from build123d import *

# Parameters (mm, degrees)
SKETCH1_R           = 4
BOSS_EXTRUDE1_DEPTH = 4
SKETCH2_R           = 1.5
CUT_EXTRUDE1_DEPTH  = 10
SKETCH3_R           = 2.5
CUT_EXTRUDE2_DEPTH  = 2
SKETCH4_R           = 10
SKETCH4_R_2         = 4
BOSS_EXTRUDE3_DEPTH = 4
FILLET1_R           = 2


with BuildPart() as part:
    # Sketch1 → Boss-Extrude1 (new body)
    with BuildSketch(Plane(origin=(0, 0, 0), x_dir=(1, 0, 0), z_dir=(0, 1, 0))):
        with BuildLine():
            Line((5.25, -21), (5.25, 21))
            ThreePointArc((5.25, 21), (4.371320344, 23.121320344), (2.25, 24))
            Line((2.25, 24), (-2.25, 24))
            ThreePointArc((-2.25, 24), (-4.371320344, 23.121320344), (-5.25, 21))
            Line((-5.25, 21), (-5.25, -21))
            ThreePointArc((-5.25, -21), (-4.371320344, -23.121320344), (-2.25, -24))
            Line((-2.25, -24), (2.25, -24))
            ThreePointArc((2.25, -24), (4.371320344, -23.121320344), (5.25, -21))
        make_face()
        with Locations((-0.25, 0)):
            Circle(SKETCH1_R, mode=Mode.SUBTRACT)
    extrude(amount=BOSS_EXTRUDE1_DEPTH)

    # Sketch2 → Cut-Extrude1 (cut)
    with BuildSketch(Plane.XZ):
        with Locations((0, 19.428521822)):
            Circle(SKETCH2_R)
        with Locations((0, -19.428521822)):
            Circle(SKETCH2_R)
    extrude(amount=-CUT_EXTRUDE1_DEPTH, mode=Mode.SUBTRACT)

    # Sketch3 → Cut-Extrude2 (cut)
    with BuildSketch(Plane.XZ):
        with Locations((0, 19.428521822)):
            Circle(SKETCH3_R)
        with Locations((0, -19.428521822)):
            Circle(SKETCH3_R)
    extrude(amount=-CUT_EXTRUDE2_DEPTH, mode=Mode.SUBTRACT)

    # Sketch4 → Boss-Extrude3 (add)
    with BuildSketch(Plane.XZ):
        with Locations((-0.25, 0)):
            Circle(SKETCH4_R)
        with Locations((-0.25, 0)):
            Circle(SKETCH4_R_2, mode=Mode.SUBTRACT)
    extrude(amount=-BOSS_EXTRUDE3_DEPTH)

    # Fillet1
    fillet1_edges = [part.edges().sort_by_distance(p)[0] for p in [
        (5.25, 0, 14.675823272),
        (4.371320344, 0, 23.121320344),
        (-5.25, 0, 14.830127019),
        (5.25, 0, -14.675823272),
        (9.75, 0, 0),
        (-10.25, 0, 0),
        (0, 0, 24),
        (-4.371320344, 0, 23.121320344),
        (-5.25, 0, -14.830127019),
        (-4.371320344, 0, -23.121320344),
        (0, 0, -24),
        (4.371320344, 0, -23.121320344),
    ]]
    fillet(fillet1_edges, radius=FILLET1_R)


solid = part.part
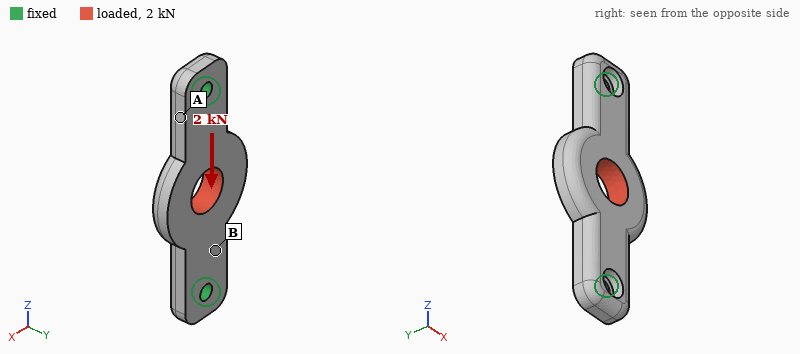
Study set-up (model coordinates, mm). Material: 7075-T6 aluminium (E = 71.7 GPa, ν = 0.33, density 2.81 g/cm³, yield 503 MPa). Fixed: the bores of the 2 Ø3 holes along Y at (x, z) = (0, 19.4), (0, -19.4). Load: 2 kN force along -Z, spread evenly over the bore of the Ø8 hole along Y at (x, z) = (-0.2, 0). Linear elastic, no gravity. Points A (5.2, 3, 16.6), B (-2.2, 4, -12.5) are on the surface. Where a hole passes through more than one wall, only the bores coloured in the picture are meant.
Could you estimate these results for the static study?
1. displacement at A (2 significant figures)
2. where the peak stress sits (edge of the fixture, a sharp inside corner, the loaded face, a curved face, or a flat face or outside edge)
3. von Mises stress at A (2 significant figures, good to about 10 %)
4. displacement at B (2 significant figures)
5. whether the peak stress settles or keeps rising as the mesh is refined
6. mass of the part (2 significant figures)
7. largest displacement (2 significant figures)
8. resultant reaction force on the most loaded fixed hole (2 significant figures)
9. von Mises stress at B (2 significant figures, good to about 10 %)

3.4 µm
edge of the fixture
16 MPa
4.6 µm
keeps rising
5.7 g
9.2 µm
1.0 kN
40 MPa
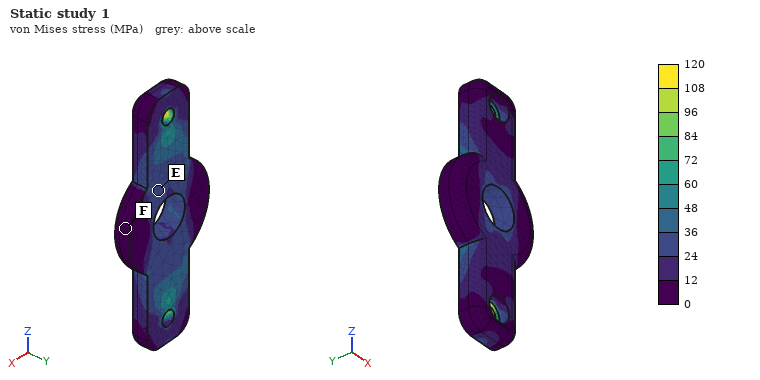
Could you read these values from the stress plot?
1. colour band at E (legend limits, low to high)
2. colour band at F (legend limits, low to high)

24 to 36 MPa
0 to 12 MPa
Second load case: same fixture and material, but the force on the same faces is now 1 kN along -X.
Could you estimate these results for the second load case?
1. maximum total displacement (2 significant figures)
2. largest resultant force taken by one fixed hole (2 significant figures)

23 µm
500 N
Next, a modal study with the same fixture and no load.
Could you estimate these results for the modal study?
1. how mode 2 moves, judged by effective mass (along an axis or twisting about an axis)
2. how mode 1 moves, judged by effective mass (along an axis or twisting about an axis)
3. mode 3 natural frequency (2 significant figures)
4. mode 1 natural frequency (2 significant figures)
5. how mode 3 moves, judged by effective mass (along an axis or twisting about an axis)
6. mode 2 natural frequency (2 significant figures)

twisting about Z
along Y
20 kHz
9000 Hz
along X
12 kHz
